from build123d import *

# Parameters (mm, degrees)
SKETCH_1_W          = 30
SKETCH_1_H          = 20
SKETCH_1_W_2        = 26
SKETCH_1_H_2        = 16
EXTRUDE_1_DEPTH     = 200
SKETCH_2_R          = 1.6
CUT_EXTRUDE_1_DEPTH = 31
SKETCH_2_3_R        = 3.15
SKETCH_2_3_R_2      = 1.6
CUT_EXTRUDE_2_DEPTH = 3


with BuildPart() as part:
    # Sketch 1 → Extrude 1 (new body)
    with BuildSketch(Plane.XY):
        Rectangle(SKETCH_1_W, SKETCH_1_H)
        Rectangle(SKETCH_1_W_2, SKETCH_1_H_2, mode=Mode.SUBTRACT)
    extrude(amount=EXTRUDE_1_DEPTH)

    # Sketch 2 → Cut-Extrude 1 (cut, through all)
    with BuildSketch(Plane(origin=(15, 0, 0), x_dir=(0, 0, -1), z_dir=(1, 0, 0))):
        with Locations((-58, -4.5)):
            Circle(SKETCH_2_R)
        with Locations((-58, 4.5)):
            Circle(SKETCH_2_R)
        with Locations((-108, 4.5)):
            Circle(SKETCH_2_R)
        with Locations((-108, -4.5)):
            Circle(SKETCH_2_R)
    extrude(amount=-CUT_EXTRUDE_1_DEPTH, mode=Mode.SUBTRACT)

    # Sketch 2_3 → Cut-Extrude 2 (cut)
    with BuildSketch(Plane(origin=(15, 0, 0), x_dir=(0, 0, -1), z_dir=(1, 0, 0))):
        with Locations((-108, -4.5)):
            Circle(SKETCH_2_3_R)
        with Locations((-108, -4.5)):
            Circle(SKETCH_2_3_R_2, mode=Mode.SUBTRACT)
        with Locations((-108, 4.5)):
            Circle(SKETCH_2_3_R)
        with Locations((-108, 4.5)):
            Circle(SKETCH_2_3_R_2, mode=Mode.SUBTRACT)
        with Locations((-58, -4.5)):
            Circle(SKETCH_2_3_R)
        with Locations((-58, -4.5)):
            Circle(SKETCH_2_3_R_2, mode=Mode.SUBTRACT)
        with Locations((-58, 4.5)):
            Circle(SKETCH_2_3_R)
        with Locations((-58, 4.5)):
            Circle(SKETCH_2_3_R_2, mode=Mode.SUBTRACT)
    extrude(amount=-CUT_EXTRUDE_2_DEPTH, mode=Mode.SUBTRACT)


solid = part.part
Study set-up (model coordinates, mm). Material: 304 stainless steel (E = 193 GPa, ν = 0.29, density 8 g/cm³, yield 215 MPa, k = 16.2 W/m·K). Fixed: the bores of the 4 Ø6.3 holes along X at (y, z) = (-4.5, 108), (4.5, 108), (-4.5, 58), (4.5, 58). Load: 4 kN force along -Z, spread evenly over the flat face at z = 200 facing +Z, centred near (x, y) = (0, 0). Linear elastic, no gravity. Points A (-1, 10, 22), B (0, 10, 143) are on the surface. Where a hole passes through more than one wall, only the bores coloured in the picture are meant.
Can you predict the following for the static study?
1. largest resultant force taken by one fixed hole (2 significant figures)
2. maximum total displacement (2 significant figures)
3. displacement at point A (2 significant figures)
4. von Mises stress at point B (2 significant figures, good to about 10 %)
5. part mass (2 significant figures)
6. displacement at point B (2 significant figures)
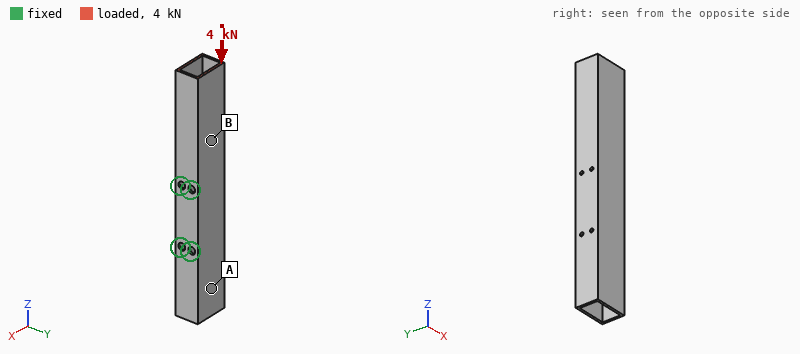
1.4 kN
39 µm
9.7 µm
21 MPa
290 g
16 µm
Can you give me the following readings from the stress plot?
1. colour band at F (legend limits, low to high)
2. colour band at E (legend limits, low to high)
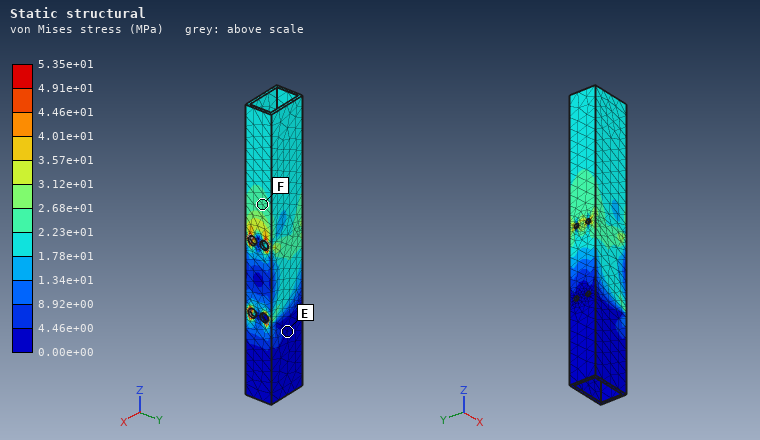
2.23e+01 to 2.68e+01 MPa
0.00e+00 to 4.46e+00 MPa
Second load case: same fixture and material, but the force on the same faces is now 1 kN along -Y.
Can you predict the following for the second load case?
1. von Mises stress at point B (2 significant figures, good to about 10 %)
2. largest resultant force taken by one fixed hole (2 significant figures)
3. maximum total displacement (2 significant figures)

51 MPa
4.0 kN
0.28 mm
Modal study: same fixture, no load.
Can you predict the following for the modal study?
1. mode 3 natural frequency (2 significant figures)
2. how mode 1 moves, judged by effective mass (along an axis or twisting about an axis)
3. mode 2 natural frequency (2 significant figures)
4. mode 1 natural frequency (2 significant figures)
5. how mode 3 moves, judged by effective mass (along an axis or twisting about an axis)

2100 Hz
along Y
1900 Hz
1400 Hz
along X
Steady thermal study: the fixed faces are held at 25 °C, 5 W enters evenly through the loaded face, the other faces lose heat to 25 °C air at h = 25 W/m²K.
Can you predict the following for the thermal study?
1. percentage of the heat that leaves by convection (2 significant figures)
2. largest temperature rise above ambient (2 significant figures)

97 %
43 K
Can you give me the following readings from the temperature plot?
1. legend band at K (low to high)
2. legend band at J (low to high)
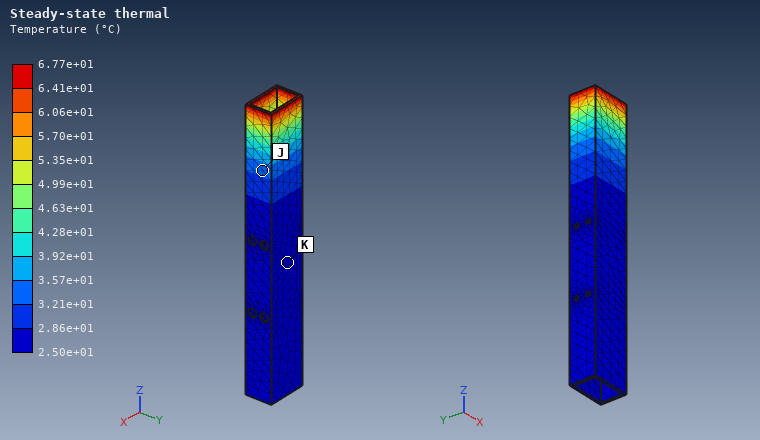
2.50e+01 to 2.86e+01 °C
3.21e+01 to 3.57e+01 °C
